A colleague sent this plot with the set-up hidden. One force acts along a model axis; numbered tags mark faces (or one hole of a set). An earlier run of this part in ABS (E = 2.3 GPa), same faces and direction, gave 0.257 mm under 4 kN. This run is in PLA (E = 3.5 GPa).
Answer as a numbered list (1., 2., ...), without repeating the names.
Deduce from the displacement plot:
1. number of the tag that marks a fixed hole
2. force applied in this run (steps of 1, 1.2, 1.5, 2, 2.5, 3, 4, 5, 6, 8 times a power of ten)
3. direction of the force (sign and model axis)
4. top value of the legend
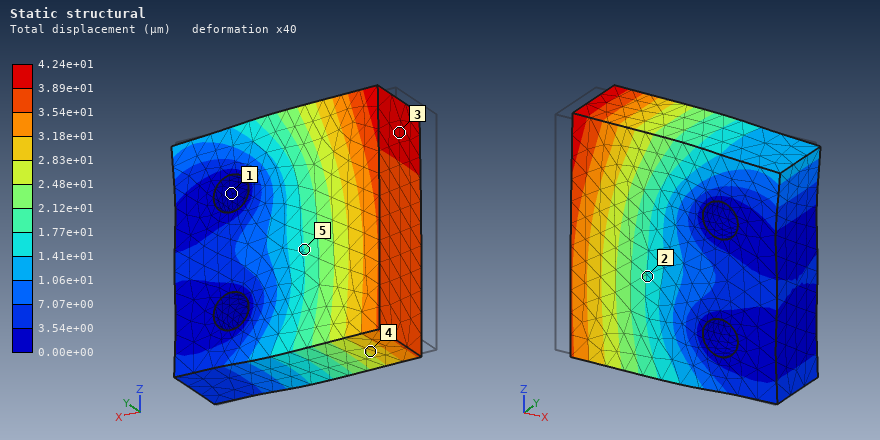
1. 1
2. 1 kN
3. +X
4. 4.24e+01 µm
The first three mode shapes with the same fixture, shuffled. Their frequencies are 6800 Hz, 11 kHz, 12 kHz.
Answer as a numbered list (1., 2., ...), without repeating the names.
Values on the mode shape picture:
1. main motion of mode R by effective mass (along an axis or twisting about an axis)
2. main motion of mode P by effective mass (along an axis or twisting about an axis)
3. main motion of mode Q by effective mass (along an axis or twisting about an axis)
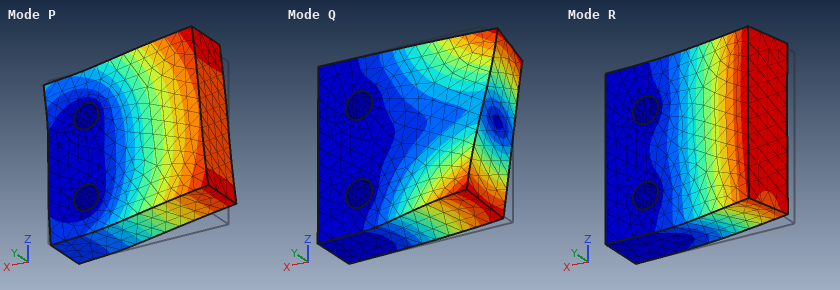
1. along Y
2. along Z
3. twisting about X
